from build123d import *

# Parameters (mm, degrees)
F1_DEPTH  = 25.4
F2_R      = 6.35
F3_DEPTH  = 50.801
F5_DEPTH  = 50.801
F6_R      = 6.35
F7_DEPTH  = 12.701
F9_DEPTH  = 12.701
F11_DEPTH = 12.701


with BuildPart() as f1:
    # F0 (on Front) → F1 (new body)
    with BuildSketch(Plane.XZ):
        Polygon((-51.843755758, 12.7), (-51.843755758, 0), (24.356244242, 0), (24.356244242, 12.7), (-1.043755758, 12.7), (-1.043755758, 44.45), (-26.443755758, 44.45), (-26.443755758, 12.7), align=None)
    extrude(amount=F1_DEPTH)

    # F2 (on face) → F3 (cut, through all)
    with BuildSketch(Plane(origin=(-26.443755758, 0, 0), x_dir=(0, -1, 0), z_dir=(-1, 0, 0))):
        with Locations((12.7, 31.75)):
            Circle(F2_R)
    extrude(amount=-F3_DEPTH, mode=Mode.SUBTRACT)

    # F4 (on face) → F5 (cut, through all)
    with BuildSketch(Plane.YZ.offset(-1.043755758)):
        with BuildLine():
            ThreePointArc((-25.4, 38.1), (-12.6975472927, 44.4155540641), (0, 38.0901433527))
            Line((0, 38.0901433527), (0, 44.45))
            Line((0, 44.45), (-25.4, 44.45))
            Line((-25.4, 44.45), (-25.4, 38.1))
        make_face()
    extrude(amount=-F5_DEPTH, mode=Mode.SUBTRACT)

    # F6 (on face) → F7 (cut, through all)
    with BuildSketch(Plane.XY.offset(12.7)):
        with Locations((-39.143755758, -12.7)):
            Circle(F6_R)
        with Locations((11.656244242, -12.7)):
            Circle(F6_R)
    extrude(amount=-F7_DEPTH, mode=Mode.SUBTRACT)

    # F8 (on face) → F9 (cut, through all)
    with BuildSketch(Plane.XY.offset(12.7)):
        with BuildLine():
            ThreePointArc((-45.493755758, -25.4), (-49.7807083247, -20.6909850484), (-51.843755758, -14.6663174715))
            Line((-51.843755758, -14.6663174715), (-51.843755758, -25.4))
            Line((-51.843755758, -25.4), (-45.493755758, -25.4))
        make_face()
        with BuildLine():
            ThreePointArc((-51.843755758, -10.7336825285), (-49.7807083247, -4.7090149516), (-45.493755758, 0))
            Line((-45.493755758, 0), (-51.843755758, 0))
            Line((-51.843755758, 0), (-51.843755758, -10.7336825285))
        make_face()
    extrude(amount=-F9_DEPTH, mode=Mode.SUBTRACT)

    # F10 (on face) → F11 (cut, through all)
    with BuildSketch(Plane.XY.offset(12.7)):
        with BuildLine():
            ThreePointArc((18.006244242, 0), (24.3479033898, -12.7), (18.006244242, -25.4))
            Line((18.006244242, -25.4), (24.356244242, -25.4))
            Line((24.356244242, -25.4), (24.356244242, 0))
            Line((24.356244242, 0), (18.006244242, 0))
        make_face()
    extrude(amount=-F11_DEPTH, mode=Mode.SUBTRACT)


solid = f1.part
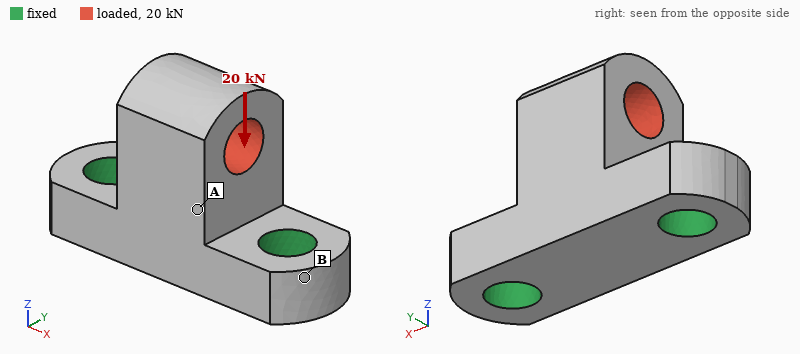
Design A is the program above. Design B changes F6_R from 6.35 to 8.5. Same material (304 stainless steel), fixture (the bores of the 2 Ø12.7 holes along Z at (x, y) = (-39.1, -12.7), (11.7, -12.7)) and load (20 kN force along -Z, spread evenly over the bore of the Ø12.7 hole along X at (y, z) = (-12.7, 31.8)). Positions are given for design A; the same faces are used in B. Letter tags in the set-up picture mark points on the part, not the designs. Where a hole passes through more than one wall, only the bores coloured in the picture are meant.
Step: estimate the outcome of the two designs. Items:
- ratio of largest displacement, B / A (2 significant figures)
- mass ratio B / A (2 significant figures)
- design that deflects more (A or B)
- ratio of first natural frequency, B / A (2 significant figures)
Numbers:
0.85
0.93
A
1.1
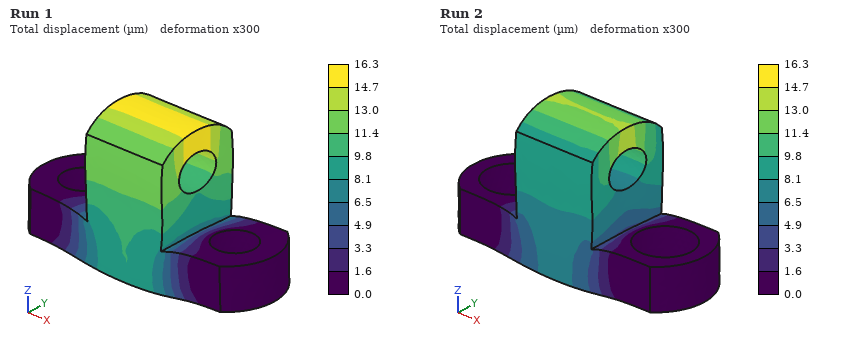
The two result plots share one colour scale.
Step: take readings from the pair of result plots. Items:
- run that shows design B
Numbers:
Run 2
